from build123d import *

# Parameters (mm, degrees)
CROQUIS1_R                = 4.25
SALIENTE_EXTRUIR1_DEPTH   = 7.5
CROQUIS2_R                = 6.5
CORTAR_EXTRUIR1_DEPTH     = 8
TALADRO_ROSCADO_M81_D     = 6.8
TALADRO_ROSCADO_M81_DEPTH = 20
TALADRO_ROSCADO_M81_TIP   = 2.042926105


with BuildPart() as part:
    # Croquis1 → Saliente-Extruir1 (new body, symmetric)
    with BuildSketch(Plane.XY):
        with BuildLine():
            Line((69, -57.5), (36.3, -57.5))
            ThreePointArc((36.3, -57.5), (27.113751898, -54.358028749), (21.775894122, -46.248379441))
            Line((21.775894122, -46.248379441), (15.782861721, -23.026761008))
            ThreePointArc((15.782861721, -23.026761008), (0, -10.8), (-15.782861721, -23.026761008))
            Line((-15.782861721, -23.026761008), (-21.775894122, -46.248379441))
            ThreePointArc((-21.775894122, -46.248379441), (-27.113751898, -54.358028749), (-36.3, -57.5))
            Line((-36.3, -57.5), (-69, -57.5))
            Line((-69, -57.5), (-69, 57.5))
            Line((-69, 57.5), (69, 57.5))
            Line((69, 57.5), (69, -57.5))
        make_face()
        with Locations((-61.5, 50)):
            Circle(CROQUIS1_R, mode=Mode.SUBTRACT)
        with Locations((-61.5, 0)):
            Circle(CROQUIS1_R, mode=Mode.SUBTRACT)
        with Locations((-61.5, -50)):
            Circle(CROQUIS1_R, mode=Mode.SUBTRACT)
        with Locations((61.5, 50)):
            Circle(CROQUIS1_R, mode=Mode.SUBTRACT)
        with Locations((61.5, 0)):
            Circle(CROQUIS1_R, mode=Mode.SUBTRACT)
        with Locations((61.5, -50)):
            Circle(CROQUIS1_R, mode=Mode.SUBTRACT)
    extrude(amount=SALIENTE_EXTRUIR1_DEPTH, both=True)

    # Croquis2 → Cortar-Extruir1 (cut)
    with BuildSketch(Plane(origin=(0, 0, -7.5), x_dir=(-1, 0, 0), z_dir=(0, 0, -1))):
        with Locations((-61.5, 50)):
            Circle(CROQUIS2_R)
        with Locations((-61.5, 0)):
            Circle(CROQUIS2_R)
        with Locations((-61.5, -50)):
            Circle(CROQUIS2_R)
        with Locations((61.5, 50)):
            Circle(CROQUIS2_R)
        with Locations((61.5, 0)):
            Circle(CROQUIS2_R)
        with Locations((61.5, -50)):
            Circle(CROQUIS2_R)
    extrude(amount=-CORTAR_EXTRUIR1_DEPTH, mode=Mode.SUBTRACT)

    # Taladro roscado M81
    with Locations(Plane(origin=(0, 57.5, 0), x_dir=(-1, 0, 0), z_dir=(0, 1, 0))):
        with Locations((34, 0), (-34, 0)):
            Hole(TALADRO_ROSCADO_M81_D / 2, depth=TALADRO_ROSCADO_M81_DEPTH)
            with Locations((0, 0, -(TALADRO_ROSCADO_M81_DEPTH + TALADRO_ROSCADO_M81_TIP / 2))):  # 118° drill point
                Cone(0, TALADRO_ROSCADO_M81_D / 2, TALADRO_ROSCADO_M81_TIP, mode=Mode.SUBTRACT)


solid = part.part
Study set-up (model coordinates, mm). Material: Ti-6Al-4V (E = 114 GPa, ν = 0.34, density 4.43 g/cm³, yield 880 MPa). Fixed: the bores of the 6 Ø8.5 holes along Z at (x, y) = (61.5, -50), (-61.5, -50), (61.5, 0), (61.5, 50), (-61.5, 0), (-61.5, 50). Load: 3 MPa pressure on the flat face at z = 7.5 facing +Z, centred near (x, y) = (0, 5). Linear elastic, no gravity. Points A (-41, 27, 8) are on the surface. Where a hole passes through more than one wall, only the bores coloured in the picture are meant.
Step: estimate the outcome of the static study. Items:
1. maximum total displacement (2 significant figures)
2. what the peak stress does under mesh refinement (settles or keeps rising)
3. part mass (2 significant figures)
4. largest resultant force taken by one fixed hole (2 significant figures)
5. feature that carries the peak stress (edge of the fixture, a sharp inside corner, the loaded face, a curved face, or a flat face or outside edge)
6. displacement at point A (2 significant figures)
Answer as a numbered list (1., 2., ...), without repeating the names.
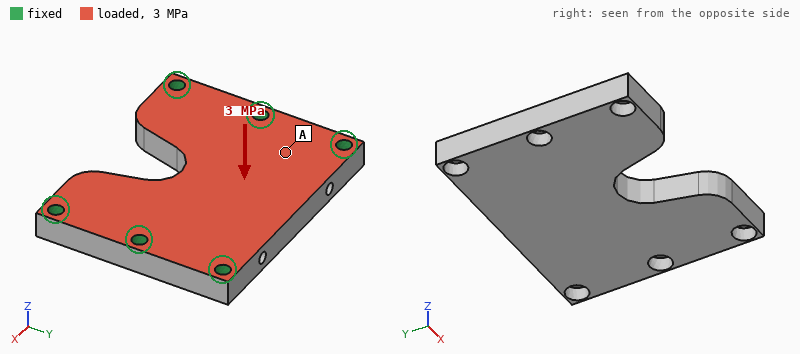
1. 0.13 mm
2. keeps rising
3. 890 g
4. 11 kN
5. edge of the fixture
6. 0.059 mm
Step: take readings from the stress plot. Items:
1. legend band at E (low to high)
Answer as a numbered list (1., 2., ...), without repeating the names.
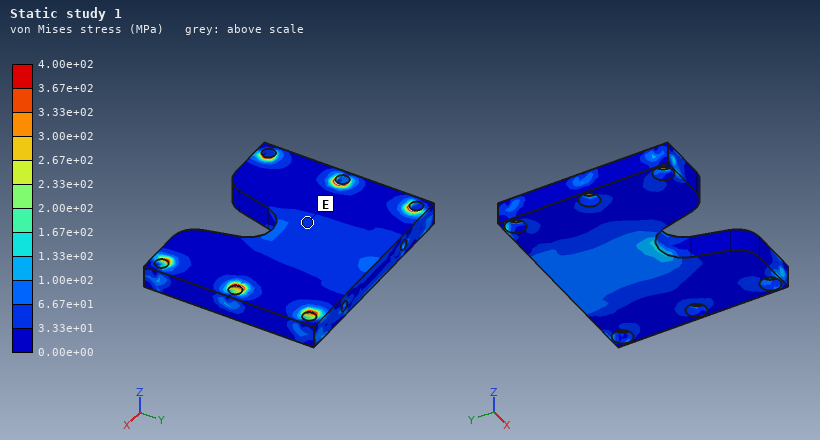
1. 3.33e+01 to 6.67e+01 MPa
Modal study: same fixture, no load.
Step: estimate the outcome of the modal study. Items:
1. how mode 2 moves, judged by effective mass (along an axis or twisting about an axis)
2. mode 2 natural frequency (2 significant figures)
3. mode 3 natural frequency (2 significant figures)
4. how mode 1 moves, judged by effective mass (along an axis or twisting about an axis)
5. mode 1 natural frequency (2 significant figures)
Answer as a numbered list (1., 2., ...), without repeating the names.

1. twisting about X
2. 5400 Hz
3. 7000 Hz
4. along Z
5. 3500 Hz
